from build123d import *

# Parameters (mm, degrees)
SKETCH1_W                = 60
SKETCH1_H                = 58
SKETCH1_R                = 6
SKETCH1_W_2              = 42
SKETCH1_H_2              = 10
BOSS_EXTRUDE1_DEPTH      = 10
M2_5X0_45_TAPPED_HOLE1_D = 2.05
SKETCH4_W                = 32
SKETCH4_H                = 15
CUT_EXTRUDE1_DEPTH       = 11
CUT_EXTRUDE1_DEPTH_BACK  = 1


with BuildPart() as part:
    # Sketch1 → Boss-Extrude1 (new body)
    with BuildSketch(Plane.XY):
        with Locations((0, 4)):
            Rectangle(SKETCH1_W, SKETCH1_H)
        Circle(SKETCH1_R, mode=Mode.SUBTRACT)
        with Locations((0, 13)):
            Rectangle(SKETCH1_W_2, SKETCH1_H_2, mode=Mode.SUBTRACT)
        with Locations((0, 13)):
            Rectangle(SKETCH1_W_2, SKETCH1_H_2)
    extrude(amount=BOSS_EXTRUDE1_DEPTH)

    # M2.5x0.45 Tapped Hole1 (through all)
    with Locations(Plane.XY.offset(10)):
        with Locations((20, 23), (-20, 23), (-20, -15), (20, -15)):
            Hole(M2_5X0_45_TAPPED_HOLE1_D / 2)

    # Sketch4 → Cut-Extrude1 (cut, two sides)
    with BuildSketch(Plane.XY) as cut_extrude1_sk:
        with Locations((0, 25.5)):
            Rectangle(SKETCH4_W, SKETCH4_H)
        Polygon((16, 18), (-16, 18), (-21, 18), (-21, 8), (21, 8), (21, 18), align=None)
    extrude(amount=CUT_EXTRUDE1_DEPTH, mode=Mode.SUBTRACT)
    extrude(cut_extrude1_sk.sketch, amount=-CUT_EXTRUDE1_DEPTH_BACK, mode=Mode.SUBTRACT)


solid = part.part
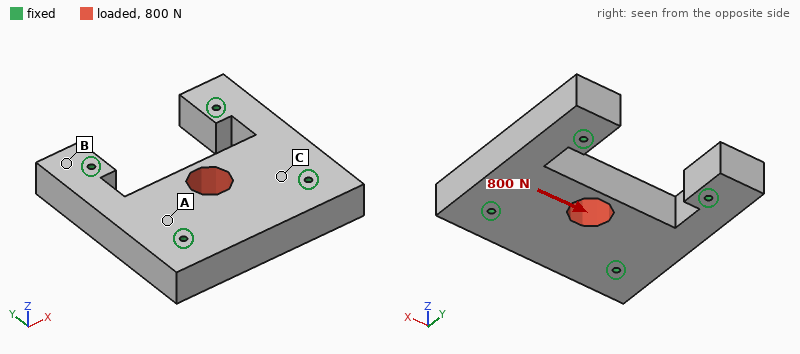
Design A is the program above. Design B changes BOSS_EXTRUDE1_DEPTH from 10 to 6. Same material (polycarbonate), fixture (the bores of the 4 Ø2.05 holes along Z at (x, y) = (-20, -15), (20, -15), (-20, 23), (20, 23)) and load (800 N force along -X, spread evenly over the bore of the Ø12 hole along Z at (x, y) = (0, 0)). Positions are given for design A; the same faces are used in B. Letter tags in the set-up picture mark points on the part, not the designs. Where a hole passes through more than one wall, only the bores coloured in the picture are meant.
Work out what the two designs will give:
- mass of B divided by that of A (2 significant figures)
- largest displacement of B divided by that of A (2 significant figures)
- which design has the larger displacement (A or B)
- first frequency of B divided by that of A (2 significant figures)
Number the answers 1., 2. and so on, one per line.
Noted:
1. 0.60
2. 1.7
3. B
4. 0.72
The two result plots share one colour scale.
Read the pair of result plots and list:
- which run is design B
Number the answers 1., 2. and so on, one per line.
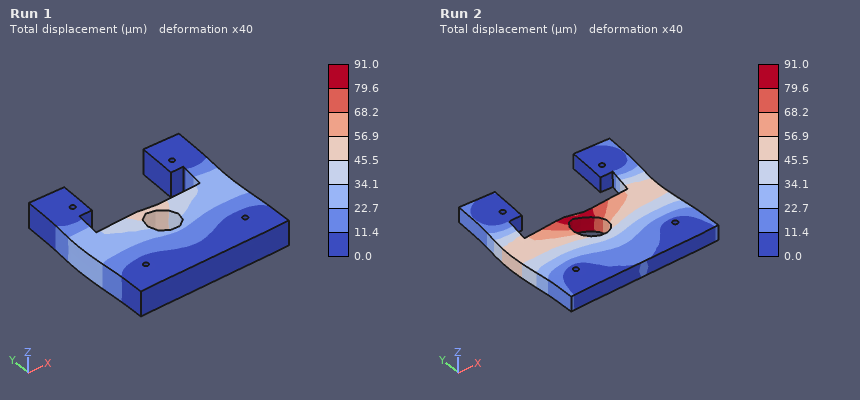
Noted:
1. Run 2
